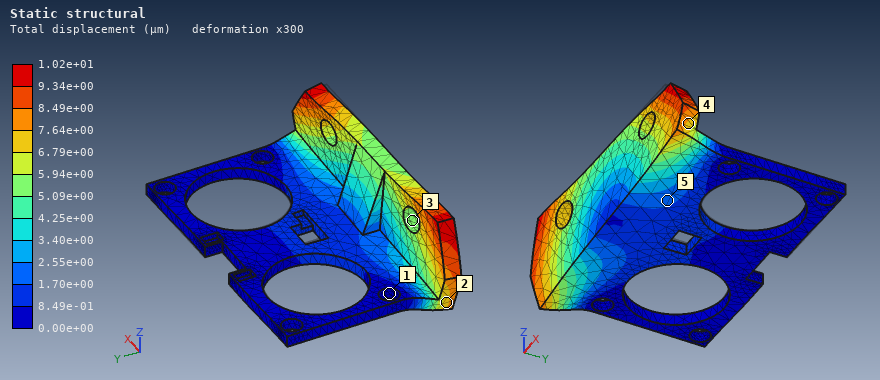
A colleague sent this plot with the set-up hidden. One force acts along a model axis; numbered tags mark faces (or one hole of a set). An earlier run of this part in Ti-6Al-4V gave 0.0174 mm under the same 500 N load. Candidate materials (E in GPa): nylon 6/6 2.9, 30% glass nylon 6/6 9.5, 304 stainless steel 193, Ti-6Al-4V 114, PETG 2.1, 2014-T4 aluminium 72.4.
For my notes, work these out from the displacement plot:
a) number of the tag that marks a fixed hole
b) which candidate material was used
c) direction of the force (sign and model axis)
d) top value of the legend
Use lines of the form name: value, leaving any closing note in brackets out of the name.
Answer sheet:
number of the tag that marks a fixed hole: 1
which candidate material was used: 304 stainless steel
direction of the force: -X
top value of the legend: 1.02e+01 µm
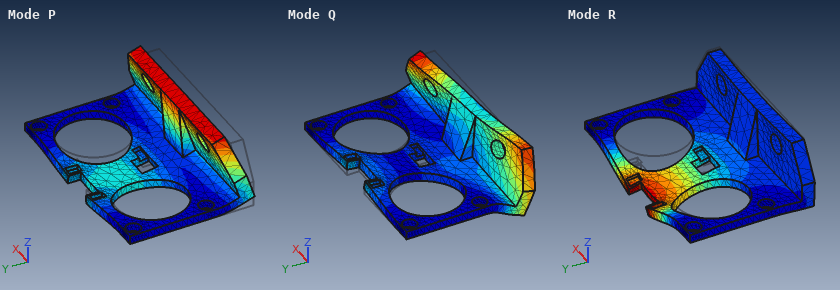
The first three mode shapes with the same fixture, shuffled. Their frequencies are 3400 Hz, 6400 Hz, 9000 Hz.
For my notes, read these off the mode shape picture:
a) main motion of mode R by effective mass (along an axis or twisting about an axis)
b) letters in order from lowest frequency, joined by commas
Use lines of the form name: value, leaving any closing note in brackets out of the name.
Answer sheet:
main motion of mode R by effective mass: along Z
letters in order from lowest frequency, joined by commas: P, R, Q
